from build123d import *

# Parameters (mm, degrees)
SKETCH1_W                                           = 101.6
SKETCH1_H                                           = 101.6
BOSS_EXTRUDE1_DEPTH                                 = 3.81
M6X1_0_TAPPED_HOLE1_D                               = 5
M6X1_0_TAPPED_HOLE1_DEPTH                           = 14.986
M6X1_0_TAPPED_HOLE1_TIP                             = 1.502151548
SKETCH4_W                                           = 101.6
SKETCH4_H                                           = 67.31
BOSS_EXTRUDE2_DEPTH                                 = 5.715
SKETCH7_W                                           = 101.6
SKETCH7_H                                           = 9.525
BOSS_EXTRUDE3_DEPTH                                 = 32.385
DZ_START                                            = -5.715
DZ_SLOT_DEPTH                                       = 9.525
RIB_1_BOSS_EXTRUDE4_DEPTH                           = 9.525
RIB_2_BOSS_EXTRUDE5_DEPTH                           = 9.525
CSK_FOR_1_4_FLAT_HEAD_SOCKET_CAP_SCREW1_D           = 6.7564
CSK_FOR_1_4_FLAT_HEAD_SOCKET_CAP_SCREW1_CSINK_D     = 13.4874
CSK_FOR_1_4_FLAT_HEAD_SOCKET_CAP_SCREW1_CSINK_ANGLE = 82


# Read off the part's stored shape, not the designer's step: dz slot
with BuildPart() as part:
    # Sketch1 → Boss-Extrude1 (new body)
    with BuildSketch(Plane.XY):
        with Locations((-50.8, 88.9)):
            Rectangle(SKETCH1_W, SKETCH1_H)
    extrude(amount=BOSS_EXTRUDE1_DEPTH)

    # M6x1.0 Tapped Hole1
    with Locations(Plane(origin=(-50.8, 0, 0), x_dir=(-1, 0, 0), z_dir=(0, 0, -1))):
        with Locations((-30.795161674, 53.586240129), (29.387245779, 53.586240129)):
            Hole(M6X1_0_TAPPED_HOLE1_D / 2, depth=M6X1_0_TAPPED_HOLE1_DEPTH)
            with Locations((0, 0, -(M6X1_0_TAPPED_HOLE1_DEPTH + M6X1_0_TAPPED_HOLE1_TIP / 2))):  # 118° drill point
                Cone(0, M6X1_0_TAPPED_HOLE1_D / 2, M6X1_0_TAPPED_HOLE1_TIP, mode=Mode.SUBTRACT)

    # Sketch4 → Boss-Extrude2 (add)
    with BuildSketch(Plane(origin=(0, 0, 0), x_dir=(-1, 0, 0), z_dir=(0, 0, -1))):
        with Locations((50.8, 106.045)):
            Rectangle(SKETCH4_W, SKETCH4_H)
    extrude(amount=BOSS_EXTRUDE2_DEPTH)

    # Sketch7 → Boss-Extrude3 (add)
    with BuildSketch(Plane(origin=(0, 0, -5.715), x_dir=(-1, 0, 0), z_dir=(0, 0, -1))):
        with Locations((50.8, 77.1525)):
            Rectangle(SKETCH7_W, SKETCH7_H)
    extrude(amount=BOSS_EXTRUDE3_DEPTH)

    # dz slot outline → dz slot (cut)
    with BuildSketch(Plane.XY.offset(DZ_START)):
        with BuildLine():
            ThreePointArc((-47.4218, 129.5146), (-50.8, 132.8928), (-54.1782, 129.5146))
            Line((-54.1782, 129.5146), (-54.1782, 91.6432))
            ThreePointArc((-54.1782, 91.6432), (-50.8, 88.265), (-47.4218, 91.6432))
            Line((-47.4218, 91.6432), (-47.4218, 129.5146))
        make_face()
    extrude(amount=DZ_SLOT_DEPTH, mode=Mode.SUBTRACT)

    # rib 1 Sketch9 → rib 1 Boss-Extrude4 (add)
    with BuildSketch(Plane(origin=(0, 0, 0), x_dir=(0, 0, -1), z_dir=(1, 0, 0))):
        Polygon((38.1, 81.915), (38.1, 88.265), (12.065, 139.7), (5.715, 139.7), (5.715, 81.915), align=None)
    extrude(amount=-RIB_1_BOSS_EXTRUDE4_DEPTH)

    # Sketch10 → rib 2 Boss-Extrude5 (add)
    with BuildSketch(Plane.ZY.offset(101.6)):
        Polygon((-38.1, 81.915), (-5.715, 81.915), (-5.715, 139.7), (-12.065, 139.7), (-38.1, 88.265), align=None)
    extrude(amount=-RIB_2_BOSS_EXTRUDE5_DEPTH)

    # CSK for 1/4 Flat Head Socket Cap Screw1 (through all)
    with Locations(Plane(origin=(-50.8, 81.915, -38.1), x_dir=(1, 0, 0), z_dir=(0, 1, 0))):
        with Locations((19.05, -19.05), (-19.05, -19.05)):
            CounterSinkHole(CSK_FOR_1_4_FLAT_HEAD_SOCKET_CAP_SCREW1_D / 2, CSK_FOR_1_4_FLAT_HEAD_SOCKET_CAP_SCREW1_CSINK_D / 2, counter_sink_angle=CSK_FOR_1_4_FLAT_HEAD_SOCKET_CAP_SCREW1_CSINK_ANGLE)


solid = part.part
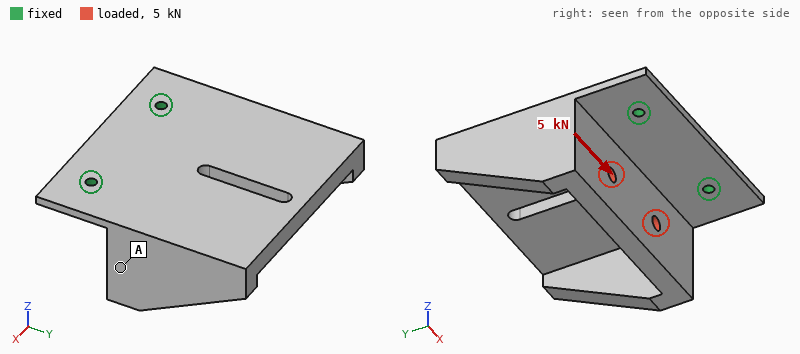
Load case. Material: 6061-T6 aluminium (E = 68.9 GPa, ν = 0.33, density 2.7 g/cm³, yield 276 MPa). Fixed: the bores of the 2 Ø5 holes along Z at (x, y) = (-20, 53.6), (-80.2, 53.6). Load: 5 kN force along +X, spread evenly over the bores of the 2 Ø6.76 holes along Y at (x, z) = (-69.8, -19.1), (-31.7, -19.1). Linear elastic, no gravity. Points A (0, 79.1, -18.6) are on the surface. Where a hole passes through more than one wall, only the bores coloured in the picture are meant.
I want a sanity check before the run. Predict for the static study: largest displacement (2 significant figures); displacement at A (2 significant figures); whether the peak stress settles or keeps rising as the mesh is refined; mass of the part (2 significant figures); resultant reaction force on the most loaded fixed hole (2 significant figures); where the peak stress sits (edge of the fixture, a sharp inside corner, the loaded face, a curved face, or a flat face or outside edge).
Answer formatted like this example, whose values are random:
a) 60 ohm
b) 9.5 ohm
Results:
a) 0.32 mm
b) 0.25 mm
c) keeps rising
d) 350 g
e) 3.4 kN
f) edge of the fixture
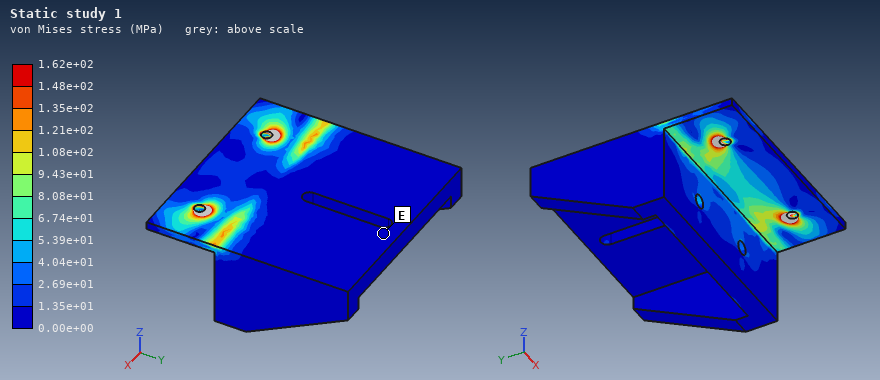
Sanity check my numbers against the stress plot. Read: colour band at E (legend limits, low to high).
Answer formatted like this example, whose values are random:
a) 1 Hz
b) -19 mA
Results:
a) 0.00e+00 to 1.35e+01 MPa
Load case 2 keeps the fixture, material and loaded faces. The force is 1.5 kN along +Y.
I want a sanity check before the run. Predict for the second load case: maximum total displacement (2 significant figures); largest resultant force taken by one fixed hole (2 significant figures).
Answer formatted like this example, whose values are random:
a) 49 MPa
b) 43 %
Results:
a) 1.7 mm
b) 770 N
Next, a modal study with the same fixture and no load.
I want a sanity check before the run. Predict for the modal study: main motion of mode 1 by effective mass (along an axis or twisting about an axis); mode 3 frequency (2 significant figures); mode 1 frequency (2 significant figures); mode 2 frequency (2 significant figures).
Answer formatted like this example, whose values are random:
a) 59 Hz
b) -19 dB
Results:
a) along Z
b) 2400 Hz
c) 240 Hz
d) 1000 Hz
